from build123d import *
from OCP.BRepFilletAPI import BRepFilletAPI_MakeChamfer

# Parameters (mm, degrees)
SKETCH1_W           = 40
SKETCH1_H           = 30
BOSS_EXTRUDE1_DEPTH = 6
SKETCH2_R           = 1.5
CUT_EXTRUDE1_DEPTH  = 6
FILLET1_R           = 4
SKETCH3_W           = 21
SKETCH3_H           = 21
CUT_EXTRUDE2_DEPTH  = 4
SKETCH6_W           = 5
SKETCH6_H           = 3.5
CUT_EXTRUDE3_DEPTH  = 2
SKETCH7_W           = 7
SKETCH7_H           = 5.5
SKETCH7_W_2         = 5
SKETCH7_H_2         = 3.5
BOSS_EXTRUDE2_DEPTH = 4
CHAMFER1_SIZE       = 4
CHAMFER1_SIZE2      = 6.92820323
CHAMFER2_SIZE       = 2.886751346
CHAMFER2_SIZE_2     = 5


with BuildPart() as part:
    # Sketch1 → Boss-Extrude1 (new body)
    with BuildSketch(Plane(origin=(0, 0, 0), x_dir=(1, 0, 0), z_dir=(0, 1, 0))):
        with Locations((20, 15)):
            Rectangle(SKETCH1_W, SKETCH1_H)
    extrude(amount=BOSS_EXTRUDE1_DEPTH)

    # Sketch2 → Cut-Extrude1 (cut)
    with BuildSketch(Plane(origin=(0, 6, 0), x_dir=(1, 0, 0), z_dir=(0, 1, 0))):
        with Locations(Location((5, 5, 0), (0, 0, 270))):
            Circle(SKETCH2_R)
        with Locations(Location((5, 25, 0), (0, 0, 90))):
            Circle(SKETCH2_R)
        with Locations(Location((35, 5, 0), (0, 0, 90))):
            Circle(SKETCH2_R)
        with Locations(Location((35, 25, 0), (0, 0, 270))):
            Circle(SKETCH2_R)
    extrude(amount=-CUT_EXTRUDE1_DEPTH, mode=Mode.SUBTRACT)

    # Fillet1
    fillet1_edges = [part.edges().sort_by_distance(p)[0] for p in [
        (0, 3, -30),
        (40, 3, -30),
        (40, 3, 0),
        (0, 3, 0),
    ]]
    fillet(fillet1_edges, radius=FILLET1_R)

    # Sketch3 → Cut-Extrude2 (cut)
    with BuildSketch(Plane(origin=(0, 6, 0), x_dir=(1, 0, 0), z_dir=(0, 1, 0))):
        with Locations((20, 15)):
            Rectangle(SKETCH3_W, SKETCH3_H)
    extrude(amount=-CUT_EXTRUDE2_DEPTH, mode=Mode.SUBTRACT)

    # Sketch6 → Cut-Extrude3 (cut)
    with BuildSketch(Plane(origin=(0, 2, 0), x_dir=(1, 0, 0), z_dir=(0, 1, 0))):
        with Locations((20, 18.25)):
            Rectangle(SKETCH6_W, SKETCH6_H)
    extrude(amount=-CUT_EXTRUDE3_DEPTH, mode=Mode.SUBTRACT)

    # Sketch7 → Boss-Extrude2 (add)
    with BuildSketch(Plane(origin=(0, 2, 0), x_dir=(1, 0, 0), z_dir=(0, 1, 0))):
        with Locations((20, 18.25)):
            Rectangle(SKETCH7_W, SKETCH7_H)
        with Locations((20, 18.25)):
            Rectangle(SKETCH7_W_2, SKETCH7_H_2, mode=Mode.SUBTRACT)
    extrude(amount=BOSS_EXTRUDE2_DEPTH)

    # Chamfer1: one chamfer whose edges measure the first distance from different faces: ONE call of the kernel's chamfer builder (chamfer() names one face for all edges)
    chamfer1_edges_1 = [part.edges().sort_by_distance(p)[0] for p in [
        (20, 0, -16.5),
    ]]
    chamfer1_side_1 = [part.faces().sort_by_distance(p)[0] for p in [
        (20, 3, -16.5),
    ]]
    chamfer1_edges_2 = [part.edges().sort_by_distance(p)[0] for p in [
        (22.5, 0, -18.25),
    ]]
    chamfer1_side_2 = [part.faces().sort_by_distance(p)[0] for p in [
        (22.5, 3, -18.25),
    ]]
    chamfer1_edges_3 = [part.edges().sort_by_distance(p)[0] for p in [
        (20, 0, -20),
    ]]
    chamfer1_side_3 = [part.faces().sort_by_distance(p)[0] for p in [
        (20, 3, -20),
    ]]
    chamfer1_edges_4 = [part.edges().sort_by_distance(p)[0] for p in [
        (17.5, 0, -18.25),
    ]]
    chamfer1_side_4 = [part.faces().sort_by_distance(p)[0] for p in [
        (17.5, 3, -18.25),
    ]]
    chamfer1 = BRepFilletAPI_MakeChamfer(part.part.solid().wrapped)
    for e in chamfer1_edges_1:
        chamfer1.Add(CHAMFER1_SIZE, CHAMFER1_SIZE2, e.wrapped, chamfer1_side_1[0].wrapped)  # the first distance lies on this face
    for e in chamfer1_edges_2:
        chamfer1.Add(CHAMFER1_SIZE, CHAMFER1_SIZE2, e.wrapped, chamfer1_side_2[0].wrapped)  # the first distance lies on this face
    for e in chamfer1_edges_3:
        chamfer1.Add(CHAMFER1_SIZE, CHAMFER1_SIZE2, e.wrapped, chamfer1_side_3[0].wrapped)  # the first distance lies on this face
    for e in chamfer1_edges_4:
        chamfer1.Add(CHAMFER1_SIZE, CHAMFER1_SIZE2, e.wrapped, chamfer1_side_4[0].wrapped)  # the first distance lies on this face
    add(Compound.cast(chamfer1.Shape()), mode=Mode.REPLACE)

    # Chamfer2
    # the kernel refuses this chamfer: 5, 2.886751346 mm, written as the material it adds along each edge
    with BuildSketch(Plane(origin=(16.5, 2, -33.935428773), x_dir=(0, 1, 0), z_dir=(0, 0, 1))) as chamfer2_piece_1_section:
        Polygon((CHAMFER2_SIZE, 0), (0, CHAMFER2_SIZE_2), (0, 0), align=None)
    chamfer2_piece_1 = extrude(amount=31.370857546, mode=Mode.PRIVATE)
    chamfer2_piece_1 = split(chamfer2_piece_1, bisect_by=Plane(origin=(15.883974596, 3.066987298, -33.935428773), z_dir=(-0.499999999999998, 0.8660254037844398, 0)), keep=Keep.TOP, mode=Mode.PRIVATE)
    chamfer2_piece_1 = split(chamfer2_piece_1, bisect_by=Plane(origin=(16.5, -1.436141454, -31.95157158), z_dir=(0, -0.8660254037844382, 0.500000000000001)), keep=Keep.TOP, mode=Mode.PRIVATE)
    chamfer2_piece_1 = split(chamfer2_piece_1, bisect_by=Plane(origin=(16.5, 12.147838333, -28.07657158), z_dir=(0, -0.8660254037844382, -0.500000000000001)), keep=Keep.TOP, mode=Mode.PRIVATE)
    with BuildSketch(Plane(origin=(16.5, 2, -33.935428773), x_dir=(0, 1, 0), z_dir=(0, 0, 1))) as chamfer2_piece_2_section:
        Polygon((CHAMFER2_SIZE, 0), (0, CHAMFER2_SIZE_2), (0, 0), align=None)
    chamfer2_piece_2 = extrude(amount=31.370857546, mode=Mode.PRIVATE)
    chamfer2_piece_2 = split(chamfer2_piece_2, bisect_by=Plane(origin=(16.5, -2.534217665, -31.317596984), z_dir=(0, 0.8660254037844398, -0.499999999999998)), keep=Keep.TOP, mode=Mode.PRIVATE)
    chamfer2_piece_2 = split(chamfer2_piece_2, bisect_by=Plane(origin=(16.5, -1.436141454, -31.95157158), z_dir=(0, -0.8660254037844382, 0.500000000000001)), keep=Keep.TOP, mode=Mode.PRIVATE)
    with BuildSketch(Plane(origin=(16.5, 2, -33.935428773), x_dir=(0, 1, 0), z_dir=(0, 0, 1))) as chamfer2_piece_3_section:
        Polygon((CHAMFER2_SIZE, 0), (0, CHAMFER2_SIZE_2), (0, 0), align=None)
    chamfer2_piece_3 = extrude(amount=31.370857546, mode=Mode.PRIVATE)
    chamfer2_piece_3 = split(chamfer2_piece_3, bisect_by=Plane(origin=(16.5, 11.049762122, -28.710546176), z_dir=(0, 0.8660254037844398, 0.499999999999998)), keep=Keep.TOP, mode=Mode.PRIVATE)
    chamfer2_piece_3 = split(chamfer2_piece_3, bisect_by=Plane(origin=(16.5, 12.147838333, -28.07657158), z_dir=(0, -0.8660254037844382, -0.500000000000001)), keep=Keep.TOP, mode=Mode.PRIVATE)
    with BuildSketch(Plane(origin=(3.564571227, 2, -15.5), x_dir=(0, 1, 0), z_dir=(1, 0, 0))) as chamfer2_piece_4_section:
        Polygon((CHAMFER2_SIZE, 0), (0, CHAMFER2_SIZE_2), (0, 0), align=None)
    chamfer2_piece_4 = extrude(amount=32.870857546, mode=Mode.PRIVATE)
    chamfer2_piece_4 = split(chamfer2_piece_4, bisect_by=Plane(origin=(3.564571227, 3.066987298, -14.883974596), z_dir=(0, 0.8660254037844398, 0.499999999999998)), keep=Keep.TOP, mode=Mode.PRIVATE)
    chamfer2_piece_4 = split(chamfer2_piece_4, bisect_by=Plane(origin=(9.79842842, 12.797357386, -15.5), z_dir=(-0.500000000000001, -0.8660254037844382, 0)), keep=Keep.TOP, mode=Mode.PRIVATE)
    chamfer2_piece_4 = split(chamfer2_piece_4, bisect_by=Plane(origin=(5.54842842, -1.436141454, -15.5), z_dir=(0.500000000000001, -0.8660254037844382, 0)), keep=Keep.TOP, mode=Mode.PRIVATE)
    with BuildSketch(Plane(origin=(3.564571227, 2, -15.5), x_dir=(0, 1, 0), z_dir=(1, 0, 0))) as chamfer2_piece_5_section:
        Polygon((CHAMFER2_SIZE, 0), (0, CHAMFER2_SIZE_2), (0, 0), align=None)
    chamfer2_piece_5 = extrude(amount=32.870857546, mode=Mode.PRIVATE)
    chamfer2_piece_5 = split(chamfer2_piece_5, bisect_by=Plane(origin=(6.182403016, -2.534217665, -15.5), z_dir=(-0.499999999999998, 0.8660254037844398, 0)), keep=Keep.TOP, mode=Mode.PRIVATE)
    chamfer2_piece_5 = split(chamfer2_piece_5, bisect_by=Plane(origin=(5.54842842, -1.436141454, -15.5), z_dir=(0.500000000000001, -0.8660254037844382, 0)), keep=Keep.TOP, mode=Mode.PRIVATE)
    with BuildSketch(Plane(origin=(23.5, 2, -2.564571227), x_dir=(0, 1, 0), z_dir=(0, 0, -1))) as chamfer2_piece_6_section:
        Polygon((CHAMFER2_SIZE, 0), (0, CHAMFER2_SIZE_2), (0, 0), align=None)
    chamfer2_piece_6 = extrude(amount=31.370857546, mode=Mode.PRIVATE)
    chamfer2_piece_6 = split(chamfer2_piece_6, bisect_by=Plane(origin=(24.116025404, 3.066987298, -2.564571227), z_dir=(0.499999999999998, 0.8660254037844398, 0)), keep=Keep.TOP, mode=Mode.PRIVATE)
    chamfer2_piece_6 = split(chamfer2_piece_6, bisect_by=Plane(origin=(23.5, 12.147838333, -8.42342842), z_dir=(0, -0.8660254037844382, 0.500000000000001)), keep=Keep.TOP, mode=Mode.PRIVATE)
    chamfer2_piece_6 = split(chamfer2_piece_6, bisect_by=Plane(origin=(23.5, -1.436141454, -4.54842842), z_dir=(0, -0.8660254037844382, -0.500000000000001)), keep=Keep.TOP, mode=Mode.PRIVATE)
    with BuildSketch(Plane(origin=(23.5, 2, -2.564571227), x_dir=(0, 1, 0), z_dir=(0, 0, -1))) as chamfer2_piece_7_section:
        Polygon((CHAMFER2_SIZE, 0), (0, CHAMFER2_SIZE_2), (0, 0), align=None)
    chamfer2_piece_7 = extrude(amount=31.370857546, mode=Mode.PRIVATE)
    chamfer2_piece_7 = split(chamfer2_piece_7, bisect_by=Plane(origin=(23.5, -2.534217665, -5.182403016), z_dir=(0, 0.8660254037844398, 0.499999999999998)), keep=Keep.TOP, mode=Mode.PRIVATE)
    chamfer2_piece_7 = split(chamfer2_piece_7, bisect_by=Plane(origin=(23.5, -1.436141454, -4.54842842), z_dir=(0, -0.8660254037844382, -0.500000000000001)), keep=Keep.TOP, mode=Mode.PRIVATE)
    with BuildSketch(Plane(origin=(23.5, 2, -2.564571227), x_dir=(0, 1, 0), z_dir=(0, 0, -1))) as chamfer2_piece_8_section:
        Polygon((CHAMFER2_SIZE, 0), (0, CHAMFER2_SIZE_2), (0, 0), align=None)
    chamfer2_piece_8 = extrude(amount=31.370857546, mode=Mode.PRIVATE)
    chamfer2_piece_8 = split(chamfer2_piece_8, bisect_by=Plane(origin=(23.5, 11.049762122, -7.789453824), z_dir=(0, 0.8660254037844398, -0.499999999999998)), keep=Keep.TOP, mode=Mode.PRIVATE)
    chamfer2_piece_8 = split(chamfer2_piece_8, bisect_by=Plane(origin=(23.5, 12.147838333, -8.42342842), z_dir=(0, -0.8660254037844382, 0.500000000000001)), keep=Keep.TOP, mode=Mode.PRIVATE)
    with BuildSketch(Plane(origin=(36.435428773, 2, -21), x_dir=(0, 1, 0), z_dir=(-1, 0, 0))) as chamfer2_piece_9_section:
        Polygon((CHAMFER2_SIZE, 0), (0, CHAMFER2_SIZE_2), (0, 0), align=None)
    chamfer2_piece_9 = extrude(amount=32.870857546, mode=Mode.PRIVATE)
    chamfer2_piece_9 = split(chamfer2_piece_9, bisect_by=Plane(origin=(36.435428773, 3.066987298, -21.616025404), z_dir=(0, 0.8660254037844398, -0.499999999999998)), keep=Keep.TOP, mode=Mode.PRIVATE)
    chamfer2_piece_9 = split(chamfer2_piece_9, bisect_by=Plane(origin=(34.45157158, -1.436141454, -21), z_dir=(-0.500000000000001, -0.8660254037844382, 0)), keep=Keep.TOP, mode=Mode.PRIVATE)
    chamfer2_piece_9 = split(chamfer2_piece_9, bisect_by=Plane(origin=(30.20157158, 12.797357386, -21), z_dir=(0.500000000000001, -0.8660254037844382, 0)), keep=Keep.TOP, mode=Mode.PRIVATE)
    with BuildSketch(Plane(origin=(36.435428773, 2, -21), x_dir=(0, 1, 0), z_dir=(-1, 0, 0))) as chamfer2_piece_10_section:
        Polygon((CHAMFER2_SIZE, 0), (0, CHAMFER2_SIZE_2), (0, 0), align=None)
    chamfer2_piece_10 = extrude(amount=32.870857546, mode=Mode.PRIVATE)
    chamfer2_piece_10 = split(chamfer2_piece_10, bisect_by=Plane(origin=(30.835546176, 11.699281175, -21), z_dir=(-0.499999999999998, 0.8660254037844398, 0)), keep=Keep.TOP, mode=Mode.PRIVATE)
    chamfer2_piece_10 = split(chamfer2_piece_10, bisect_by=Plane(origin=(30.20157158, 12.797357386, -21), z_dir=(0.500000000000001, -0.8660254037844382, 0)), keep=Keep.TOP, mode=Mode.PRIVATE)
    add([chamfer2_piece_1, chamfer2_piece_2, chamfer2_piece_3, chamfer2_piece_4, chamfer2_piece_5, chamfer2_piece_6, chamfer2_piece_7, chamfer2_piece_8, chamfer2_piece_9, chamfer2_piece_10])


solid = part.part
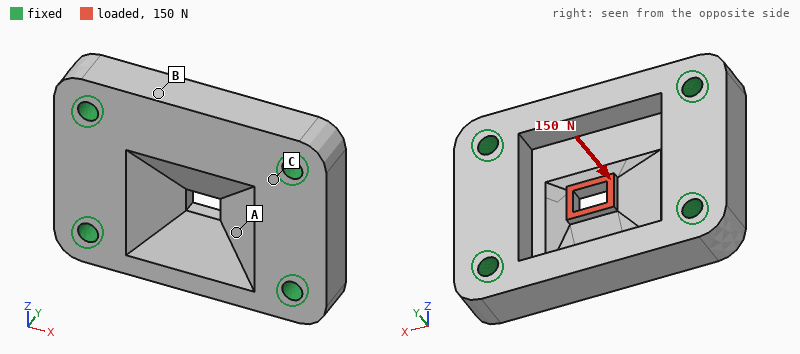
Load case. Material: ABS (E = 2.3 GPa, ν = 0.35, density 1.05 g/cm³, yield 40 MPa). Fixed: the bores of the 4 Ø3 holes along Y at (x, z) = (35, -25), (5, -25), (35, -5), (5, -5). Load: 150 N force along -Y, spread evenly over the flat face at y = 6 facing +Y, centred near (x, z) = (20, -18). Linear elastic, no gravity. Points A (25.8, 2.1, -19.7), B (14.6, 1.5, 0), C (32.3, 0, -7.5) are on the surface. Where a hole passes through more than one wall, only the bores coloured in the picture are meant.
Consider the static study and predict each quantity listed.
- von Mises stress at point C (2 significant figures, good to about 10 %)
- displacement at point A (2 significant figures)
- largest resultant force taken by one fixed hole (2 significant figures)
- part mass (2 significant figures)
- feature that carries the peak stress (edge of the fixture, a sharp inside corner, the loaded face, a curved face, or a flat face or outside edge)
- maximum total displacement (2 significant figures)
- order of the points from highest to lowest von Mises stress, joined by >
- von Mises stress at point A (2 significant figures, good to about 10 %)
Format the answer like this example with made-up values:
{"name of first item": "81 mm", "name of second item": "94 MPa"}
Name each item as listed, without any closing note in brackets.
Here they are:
{"von Mises stress at point C": "5.4 MPa", "displacement at point A": "0.090 mm", "largest resultant force taken by one fixed hole": "68 N", "part mass": "5.3 g", "feature that carries the peak stress": "the loaded face", "maximum total displacement": "0.16 mm", "order of the points from highest to lowest von Mises stress, joined by >": "A > C > B", "von Mises stress at point A": "9.1 MPa"}
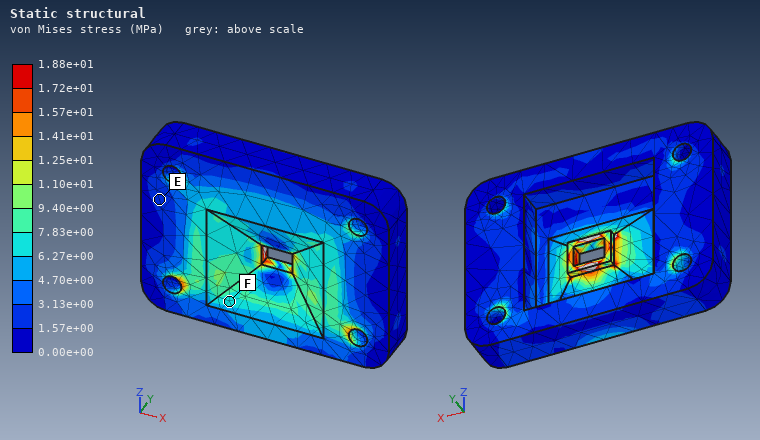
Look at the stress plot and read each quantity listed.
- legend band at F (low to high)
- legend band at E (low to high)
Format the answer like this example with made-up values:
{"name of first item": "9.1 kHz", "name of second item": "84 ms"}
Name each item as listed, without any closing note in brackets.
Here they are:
{"legend band at F": "6.27e+00 to 7.83e+00 MPa", "legend band at E": "1.57e+00 to 3.13e+00 MPa"}
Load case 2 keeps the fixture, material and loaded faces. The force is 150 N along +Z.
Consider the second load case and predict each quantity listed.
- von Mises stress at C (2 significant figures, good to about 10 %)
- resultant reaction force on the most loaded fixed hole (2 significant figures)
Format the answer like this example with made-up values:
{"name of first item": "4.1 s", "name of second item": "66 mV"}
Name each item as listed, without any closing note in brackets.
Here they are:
{"von Mises stress at C": "4.4 MPa", "resultant reaction force on the most loaded fixed hole": "46 N"}
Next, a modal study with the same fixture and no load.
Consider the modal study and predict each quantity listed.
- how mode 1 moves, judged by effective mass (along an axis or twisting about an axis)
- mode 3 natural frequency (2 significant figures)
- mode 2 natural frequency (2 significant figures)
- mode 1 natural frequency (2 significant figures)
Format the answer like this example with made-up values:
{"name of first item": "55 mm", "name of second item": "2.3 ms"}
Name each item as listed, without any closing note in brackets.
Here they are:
{"how mode 1 moves, judged by effective mass": "along Y", "mode 3 natural frequency": "10 kHz", "mode 2 natural frequency": "8800 Hz", "mode 1 natural frequency": "7800 Hz"}
